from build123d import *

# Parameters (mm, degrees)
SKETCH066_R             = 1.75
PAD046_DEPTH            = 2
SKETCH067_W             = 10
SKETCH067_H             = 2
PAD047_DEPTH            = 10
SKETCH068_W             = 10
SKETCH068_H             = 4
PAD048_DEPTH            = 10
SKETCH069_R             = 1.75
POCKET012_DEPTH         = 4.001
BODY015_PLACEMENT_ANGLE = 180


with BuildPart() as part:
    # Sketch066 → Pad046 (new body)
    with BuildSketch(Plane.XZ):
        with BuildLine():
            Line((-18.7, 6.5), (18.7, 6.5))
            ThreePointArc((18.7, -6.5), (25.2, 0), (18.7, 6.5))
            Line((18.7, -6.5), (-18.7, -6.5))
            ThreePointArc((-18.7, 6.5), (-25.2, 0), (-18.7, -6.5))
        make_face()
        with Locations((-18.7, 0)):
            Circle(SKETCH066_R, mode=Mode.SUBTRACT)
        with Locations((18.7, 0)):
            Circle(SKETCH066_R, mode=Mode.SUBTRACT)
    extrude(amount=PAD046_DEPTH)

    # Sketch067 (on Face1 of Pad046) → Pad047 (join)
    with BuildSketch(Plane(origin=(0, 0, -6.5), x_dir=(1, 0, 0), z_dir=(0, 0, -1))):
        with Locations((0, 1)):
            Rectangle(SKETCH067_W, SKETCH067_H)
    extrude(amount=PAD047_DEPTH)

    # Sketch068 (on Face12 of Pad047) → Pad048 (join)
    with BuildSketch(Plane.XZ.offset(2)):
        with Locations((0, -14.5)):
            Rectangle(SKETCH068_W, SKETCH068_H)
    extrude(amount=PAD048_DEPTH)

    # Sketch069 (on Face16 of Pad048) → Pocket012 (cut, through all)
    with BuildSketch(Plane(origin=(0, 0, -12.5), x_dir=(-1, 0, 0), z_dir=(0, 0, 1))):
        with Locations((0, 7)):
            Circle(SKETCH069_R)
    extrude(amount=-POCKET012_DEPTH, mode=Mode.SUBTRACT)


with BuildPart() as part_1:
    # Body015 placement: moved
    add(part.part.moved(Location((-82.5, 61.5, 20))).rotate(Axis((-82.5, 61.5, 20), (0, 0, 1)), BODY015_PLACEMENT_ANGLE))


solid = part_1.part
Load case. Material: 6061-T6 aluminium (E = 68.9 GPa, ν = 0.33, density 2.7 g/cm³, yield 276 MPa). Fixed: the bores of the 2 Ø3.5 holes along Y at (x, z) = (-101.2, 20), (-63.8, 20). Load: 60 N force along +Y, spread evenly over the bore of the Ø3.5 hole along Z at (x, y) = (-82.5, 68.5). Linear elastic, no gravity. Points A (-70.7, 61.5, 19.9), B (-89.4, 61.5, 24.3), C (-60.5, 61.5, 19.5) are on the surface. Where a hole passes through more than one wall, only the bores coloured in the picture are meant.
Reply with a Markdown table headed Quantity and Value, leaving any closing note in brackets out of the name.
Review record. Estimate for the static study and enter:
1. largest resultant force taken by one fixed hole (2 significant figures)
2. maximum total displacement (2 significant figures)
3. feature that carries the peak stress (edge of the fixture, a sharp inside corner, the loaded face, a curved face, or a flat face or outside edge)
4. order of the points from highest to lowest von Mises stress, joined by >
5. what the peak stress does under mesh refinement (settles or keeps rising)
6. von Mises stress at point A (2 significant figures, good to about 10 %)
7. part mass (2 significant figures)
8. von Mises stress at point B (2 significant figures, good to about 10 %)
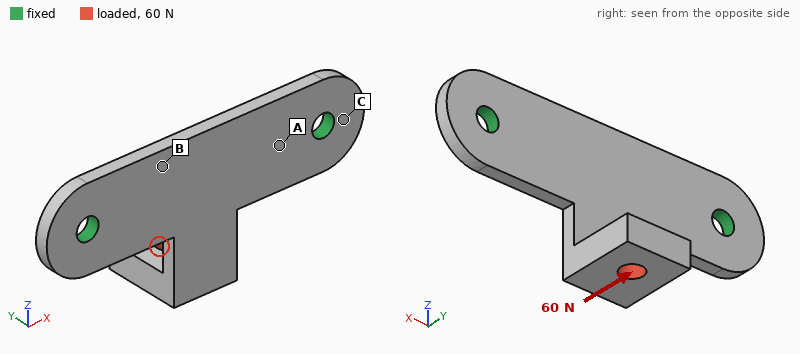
| Quantity | Value |
|---|---|
| largest resultant force taken by one fixed hole | 30 N |
| maximum total displacement | 0.27 mm |
| feature that carries the peak stress | a sharp inside corner |
| order of the points from highest to lowest von Mises stress, joined by > | A > B > C |
| what the peak stress does under mesh refinement | keeps rising |
| von Mises stress at point A | 44 MPa |
| part mass | 4.8 g |
| von Mises stress at point B | 24 MPa |
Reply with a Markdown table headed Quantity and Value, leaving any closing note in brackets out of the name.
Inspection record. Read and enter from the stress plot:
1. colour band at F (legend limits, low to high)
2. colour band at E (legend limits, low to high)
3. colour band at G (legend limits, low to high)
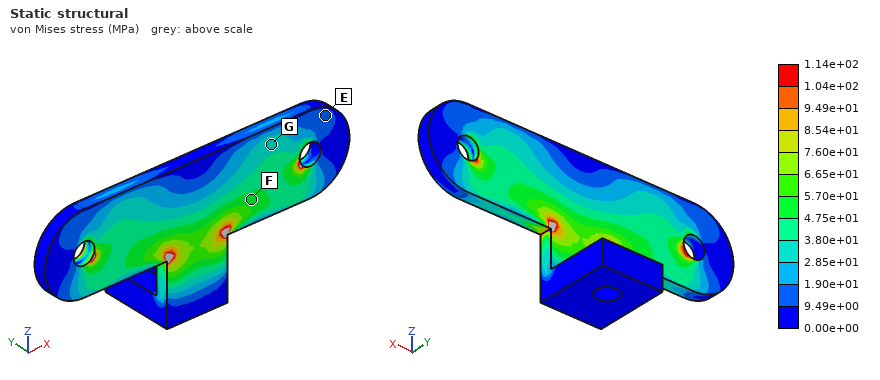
| Quantity | Value |
|---|---|
| colour band at F | 4.75e+01 to 5.70e+01 MPa |
| colour band at E | 9.49e+00 to 1.90e+01 MPa |
| colour band at G | 2.85e+01 to 3.80e+01 MPa |
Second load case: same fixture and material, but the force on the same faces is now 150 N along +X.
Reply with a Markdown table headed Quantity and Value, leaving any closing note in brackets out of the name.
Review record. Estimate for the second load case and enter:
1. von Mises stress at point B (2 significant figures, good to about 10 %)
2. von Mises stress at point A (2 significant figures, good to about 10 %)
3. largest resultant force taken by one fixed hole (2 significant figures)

| Quantity | Value |
|---|---|
| von Mises stress at point B | 14 MPa |
| von Mises stress at point A | 21 MPa |
| largest resultant force taken by one fixed hole | 110 N |
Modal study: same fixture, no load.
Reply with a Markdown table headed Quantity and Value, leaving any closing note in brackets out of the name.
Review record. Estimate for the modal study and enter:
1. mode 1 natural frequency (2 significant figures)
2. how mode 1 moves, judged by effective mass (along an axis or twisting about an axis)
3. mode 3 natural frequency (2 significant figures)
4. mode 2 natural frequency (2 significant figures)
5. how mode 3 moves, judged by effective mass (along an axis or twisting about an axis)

| Quantity | Value |
|---|---|
| mode 1 natural frequency | 2200 Hz |
| how mode 1 moves, judged by effective mass | along Y |
| mode 3 natural frequency | 6600 Hz |
| mode 2 natural frequency | 5600 Hz |
| how mode 3 moves, judged by effective mass | along Y |
